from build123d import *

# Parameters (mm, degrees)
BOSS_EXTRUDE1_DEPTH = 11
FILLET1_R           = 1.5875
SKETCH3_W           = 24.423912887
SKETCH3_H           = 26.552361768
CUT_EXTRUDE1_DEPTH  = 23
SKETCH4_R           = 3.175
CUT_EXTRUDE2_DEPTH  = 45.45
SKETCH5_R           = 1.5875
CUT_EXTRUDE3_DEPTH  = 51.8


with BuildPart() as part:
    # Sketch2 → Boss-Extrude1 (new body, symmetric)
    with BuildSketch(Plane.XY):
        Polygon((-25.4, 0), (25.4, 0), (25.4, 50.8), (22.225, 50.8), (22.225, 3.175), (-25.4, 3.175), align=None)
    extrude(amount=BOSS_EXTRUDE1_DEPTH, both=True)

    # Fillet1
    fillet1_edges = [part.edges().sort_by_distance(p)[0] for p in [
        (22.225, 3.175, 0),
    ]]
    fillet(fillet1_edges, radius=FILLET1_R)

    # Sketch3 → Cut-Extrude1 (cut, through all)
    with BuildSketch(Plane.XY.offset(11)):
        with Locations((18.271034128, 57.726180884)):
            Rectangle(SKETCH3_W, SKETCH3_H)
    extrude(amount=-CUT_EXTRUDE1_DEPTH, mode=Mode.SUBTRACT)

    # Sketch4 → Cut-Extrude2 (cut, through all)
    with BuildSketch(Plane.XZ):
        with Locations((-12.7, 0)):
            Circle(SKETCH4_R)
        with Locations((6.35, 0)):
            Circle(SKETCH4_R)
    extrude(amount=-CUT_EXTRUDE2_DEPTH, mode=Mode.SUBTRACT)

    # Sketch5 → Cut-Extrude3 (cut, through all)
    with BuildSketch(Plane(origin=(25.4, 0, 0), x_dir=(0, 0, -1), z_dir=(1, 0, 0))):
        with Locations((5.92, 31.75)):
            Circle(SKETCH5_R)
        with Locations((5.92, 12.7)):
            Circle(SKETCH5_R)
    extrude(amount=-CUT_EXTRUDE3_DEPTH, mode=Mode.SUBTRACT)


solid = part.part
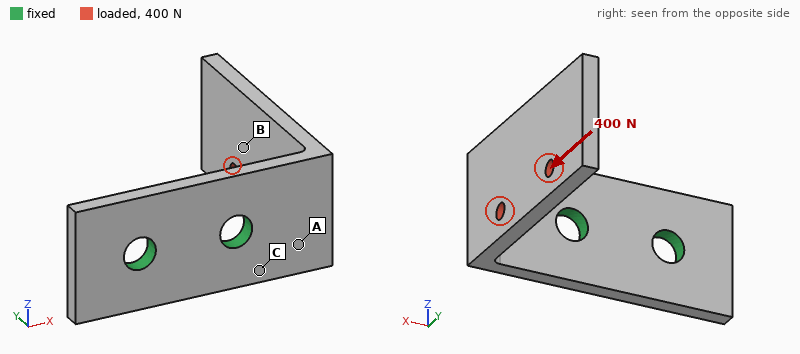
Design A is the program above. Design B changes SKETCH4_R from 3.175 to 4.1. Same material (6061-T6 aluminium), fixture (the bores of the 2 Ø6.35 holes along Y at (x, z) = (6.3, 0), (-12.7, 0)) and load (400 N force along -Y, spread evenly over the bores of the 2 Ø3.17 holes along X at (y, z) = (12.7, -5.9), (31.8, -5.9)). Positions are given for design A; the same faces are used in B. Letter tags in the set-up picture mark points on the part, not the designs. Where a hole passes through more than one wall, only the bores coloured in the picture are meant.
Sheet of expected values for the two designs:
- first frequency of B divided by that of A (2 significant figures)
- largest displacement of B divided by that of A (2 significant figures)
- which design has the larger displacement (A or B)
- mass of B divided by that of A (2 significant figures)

1.0
0.86
A
0.98
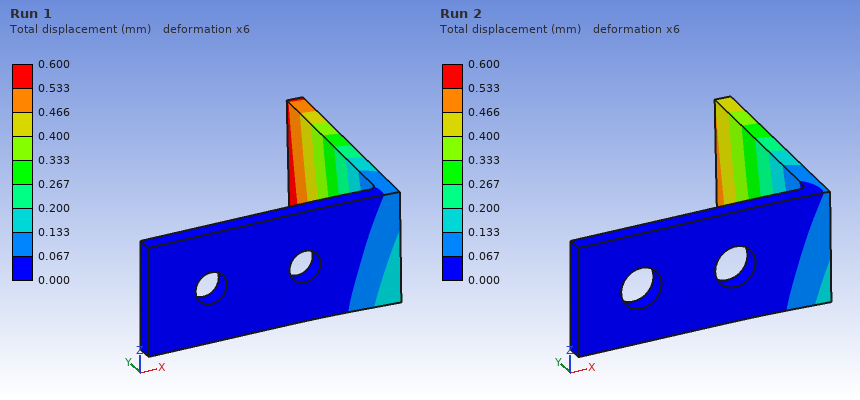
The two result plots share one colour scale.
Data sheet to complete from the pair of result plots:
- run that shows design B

Run 2
